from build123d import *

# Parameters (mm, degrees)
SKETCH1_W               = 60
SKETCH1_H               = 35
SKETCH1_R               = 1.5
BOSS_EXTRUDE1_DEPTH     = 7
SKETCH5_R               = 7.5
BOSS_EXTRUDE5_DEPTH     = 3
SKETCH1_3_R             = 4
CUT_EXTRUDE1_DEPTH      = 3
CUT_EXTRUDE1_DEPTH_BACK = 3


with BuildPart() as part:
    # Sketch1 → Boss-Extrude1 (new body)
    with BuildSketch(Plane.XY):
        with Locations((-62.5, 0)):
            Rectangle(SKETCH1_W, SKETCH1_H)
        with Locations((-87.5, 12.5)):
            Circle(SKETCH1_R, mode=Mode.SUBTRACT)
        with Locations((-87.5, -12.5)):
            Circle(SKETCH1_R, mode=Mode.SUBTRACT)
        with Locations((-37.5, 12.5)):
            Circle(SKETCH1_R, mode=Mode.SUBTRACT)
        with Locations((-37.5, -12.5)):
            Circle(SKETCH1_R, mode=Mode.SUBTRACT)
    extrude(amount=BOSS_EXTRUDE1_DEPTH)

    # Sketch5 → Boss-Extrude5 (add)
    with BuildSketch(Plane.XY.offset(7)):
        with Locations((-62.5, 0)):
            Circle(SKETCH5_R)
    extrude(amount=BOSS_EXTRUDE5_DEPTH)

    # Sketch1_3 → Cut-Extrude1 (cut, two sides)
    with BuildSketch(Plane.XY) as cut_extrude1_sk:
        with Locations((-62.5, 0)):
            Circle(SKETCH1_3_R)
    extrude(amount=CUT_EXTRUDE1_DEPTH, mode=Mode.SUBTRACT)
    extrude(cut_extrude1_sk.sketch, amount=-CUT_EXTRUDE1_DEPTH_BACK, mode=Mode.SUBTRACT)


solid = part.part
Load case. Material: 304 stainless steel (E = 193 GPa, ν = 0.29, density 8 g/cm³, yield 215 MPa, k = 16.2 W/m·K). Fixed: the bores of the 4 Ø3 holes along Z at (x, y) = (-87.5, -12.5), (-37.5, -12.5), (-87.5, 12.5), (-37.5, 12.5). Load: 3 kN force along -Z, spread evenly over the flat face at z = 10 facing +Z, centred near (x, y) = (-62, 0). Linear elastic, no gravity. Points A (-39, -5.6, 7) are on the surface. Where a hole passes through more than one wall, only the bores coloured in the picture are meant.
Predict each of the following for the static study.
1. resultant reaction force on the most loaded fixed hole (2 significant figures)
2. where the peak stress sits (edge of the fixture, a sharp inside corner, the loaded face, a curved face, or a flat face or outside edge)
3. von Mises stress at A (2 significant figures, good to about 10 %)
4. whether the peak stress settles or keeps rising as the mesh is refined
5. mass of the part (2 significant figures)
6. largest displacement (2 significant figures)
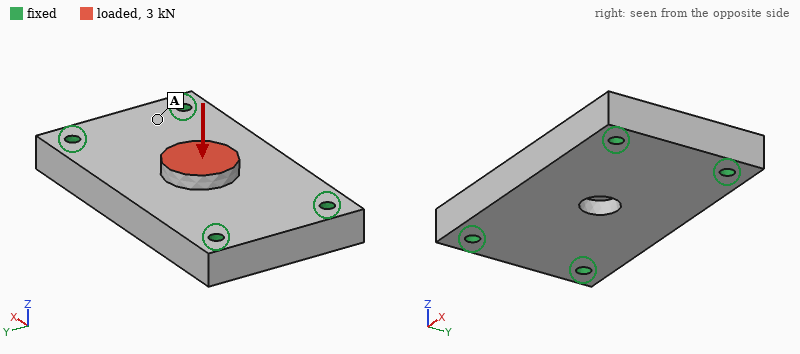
770 N
edge of the fixture
21 MPa
keeps rising
120 g
14 µm
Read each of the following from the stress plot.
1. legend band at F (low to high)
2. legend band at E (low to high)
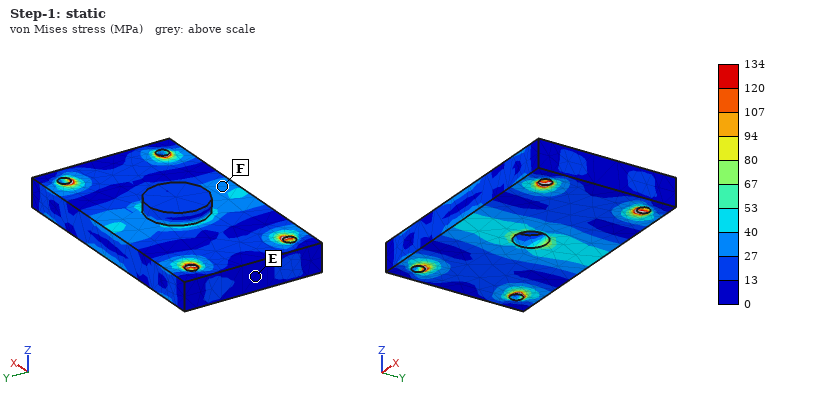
27 to 40 MPa
0 to 13 MPa
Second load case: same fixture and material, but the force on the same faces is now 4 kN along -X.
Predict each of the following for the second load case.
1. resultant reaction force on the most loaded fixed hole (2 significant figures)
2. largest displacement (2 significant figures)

1.1 kN
6.5 µm
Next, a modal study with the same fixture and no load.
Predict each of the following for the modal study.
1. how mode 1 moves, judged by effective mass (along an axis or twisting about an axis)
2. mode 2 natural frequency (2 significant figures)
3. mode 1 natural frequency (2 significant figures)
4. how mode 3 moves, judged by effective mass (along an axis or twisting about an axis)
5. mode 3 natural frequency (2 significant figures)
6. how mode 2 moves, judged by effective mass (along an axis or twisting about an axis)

along Z
16 kHz
11 kHz
along Y
24 kHz
twisting about X
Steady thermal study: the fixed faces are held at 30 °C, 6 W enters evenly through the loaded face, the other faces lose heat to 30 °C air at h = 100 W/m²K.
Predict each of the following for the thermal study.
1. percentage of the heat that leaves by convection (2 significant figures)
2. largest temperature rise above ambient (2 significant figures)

48 %
24 K
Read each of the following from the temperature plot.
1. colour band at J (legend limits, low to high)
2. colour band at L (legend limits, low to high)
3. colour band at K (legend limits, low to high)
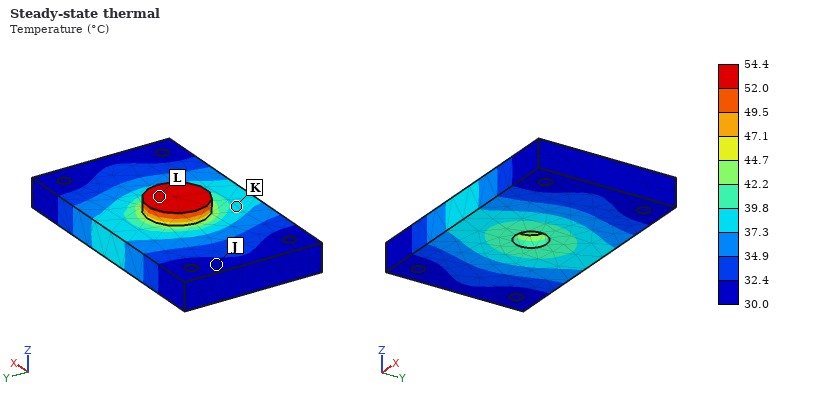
30.0 to 32.4 °C
52.0 to 54.4 °C
37.3 to 39.8 °C
